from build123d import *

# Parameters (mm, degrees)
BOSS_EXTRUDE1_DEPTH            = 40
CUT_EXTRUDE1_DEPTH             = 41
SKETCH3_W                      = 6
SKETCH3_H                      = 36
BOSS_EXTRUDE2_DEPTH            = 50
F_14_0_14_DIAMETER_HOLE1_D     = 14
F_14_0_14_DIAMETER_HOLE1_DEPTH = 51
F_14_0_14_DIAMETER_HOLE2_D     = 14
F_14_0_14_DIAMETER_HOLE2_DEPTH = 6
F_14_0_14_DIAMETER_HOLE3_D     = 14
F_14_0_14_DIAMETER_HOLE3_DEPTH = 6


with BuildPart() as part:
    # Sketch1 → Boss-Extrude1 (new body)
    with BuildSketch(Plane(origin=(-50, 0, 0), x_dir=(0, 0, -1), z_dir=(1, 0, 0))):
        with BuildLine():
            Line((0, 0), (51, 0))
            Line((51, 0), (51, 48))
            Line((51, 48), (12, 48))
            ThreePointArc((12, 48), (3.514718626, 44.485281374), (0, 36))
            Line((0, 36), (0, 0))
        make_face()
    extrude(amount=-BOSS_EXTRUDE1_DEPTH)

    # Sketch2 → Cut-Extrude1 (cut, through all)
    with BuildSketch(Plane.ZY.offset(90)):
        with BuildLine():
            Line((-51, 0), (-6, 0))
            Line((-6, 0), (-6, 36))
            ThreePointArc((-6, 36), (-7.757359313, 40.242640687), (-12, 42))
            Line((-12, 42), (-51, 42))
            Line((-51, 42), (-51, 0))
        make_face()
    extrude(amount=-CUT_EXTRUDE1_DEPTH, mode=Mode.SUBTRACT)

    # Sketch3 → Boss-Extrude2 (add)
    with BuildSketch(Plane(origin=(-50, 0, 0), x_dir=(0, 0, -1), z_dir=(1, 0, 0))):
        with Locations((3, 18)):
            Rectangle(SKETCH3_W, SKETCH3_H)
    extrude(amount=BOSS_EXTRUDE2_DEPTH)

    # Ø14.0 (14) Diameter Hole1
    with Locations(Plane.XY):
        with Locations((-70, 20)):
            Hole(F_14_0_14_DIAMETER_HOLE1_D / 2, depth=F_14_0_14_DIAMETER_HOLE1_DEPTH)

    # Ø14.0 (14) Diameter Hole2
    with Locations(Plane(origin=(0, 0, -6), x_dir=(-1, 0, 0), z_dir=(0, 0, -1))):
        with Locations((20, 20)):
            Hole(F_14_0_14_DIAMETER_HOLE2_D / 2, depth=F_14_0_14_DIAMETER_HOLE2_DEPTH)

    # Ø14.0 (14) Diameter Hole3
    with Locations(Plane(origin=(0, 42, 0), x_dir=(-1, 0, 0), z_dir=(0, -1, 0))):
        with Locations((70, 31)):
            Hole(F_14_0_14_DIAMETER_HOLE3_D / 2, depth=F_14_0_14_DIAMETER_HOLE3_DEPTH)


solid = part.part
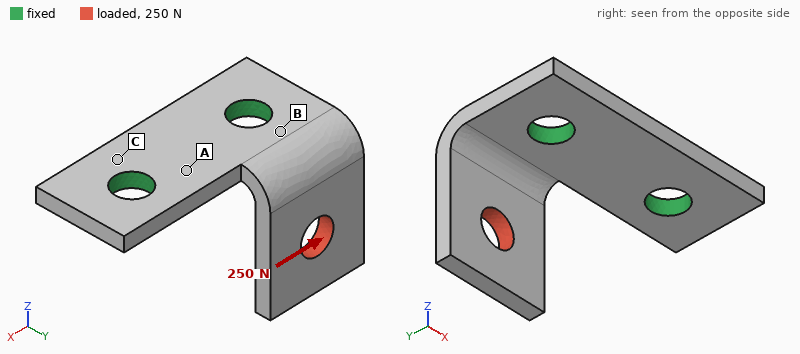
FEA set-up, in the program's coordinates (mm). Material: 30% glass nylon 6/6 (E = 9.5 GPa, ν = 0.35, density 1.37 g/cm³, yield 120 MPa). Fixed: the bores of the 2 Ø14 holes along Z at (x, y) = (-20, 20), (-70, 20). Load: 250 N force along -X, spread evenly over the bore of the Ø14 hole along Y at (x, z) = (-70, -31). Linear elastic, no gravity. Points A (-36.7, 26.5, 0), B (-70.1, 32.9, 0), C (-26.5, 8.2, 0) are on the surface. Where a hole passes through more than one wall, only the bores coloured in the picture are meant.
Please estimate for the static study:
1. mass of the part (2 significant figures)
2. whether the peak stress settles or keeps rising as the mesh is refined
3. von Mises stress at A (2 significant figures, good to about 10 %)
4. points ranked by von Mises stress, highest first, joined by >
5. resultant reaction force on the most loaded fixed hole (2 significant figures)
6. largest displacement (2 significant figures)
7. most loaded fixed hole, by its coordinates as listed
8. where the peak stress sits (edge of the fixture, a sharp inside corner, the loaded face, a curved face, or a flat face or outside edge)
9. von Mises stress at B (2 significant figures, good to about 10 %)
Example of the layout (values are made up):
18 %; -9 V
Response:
40 g; keeps rising; 6.2 MPa; B > A > C; 210 N; 0.44 mm; (-70, 20); a sharp inside corner; 12 MPa
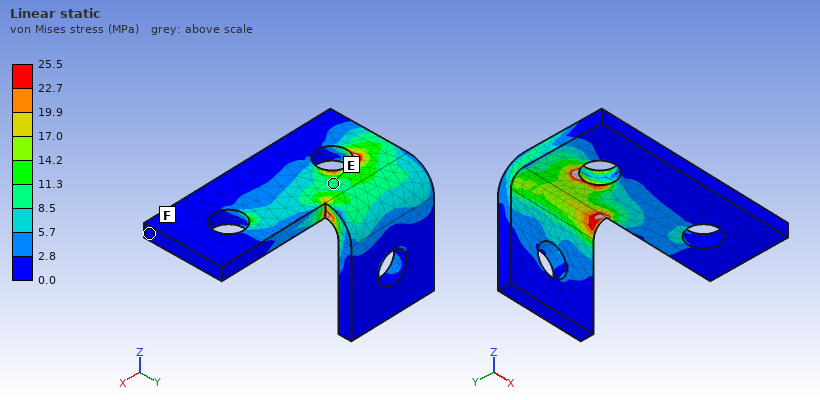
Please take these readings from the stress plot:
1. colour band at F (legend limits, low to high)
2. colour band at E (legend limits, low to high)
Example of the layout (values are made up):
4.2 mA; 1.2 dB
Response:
0.0 to 2.8 MPa; 8.5 to 11.3 MPa
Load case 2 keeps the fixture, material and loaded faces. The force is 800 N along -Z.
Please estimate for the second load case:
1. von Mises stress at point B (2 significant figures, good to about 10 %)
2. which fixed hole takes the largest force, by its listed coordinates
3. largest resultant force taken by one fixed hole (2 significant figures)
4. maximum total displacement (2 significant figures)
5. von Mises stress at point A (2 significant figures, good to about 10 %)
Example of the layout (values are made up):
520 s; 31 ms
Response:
46 MPa; (-70, 20); 800 N; 1.2 mm; 8.9 MPa
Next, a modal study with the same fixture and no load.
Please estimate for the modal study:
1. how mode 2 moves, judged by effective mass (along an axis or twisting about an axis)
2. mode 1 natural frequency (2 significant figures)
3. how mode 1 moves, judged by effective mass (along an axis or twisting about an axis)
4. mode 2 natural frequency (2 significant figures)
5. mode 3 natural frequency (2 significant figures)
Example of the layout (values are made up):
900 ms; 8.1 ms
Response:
along X; 740 Hz; along Y; 1300 Hz; 2600 Hz
